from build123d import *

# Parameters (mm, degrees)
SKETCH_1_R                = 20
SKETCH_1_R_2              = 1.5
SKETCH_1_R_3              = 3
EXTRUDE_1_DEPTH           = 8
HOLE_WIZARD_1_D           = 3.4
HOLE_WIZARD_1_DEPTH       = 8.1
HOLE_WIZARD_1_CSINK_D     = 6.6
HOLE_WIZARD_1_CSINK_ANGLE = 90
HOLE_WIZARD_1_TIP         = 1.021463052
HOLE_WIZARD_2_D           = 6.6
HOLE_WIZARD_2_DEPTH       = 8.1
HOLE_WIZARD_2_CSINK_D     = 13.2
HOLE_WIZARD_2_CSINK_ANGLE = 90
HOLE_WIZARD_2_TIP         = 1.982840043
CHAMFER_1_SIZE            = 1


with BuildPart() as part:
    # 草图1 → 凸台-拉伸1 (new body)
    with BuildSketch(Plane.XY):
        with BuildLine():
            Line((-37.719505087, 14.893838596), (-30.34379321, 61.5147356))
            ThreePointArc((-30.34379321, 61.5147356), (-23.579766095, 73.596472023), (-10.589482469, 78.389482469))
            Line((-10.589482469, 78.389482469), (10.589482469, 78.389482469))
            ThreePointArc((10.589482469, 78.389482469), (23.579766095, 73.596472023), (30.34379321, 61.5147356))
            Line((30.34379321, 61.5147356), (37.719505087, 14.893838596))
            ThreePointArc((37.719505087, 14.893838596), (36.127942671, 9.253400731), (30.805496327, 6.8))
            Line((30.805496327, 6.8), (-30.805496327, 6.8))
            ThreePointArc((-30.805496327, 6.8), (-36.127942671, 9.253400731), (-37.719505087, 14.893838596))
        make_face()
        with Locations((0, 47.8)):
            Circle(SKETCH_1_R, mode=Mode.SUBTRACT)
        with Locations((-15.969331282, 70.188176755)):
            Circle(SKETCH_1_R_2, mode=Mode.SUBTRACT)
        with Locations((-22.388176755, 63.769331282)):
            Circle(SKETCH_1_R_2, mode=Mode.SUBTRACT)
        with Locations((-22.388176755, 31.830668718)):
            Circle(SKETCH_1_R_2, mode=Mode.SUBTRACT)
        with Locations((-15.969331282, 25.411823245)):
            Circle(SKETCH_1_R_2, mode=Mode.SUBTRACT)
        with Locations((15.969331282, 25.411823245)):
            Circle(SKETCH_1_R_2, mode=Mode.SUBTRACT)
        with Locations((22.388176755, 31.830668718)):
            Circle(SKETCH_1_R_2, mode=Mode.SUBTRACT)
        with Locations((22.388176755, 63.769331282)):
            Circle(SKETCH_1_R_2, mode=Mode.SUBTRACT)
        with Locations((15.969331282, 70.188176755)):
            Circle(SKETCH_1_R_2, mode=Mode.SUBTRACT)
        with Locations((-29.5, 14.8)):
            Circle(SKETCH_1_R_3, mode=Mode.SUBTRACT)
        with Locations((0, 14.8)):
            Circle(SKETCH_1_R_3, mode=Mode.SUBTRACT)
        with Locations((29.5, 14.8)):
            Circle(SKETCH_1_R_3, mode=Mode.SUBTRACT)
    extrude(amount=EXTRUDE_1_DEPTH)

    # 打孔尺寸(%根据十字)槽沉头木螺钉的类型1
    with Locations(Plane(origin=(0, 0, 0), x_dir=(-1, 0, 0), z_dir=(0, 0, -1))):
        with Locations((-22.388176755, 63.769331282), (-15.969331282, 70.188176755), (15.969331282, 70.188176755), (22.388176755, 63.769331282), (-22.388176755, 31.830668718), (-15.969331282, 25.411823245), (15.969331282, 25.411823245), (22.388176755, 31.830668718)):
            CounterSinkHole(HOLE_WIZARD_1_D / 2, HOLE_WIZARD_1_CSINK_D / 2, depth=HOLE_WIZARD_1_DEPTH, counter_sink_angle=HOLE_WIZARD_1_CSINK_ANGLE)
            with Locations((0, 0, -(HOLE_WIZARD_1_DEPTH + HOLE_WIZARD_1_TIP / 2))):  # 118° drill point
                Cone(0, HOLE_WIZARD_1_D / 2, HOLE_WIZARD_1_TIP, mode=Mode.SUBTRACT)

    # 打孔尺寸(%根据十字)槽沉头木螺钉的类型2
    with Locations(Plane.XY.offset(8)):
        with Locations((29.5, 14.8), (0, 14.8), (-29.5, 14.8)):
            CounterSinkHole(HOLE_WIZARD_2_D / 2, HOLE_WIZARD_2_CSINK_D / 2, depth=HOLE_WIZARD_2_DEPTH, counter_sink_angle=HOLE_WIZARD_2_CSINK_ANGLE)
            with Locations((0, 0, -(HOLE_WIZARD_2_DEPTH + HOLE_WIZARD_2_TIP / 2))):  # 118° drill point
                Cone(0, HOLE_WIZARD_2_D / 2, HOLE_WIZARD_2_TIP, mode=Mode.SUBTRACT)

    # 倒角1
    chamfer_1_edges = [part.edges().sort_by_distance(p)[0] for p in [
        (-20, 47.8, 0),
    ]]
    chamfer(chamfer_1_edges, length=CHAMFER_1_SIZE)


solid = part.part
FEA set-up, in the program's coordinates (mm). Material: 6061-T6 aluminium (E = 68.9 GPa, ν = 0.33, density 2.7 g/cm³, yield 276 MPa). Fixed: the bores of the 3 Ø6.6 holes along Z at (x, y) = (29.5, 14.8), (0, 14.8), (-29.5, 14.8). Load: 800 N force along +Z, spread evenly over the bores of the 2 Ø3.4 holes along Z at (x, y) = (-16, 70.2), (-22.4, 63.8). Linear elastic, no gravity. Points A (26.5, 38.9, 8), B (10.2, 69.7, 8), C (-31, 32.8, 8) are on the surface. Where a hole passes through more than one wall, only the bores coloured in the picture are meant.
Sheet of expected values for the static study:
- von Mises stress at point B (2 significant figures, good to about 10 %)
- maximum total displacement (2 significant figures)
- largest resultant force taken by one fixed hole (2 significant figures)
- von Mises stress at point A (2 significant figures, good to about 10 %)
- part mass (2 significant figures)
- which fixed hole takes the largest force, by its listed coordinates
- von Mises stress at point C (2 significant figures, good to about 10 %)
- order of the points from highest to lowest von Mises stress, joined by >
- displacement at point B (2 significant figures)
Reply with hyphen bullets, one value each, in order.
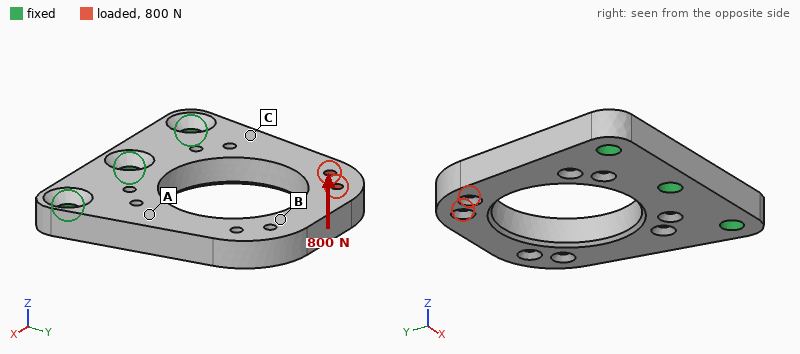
- 25 MPa
- 0.58 mm
- 540 N
- 63 MPa
- 67 g
- (-29.5, 14.8)
- 91 MPa
- C > A > B
- 0.37 mm
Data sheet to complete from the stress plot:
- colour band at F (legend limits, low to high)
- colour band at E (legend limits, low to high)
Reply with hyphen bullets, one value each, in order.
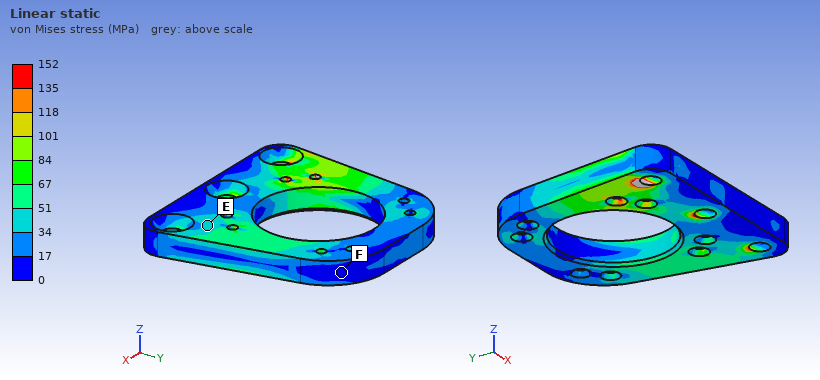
- 0 to 17 MPa
- 34 to 51 MPa
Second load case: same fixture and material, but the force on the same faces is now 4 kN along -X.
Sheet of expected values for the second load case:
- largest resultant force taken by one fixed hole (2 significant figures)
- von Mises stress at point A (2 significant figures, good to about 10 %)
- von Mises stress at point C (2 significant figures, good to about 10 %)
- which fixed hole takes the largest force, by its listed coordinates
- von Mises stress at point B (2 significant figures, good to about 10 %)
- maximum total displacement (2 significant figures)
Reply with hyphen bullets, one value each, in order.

- 3.6 kN
- 25 MPa
- 48 MPa
- (-29.5, 14.8)
- 39 MPa
- 0.14 mm
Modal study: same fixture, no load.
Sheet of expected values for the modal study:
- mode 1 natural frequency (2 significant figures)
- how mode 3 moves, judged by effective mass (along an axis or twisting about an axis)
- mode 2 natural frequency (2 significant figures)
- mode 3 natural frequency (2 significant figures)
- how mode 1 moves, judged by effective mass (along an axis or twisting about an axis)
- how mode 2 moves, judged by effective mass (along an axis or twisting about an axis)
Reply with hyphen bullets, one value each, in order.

- 1500 Hz
- along X
- 3700 Hz
- 6400 Hz
- along Z
- twisting about Y
